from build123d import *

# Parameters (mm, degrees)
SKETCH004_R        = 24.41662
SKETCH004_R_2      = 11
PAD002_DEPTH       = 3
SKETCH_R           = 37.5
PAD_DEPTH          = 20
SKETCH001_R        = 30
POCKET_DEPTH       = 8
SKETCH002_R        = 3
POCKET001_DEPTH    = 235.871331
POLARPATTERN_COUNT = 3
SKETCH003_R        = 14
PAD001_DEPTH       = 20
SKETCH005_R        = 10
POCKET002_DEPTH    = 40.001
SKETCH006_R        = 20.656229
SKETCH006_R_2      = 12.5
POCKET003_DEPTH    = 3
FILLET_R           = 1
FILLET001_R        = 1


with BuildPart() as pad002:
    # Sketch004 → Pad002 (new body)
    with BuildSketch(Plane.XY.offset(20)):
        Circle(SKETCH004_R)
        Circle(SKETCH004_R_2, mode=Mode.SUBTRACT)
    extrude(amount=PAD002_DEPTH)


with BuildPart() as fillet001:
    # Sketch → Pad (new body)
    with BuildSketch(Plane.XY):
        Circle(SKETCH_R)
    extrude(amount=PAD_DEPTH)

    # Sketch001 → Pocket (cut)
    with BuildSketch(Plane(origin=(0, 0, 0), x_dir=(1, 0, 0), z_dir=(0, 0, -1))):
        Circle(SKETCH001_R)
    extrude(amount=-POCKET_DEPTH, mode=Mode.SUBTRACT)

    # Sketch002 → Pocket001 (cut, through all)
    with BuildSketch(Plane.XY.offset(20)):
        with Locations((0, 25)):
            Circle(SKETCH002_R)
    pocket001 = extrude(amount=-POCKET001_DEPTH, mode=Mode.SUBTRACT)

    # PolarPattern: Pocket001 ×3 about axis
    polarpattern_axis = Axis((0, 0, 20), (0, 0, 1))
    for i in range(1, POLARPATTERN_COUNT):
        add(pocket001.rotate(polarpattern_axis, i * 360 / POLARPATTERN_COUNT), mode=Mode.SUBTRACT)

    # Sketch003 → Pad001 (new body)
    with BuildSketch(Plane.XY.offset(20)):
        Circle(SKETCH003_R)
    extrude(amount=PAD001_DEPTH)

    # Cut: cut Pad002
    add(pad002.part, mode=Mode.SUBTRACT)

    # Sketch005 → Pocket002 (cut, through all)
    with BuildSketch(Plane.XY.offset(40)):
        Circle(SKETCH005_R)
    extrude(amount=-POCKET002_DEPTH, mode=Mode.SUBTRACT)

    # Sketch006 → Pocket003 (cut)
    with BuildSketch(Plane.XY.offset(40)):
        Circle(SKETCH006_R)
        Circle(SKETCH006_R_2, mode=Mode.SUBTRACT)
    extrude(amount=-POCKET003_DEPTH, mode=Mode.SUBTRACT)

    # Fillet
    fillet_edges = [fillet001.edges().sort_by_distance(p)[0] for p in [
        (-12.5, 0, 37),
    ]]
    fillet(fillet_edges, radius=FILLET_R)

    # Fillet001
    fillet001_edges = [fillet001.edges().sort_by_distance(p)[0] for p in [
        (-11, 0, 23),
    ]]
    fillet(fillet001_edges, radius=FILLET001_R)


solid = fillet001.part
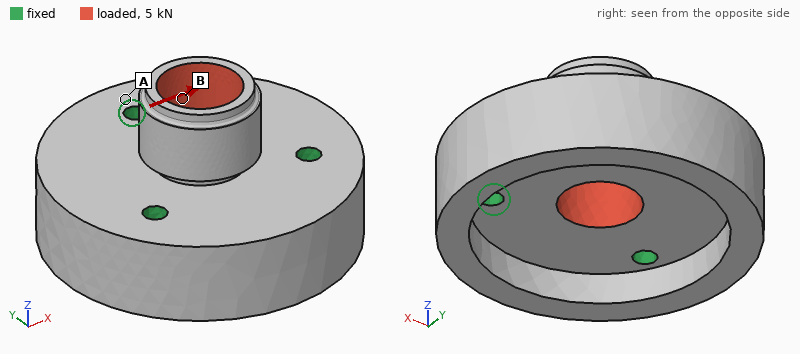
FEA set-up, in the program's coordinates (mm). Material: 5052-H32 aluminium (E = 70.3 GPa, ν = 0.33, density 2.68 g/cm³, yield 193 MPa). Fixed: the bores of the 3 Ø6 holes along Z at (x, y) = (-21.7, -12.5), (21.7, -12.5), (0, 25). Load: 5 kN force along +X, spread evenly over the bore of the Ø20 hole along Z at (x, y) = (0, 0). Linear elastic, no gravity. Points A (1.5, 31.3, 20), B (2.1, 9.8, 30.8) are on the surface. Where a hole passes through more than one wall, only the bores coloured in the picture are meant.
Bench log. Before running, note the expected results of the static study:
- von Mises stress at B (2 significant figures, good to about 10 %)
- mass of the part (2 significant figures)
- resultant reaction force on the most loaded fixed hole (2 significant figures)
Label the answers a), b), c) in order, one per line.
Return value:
a) 25 MPa
b) 180 g
c) 2.0 kN
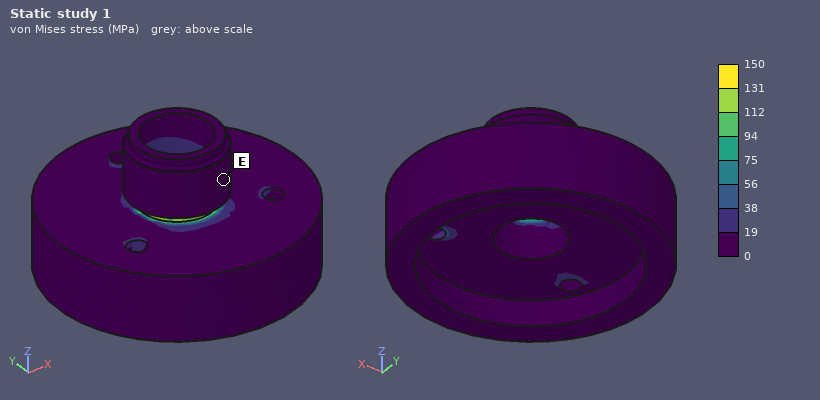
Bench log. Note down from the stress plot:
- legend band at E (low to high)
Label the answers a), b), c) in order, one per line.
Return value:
a) 0 to 19 MPa
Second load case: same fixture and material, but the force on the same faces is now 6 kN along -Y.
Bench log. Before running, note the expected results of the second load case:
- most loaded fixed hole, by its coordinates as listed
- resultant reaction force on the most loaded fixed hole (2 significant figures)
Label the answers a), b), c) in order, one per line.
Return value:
a) (0, 25)
b) 2.5 kN
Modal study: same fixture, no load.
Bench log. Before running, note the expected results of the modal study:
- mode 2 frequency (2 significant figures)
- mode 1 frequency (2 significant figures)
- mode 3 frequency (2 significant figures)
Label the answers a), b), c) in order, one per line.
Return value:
a) 11 kHz
b) 11 kHz
c) 12 kHz
